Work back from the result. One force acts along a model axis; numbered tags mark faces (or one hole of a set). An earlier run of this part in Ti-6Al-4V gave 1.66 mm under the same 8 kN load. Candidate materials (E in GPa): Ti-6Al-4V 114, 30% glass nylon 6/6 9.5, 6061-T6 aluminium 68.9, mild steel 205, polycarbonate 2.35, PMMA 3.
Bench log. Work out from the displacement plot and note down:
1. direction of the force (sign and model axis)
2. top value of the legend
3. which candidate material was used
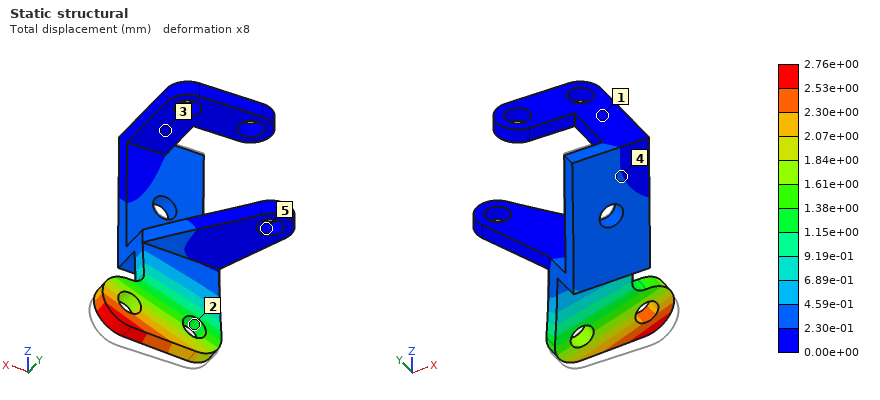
+Y
2.76e+00 mm
6061-T6 aluminium
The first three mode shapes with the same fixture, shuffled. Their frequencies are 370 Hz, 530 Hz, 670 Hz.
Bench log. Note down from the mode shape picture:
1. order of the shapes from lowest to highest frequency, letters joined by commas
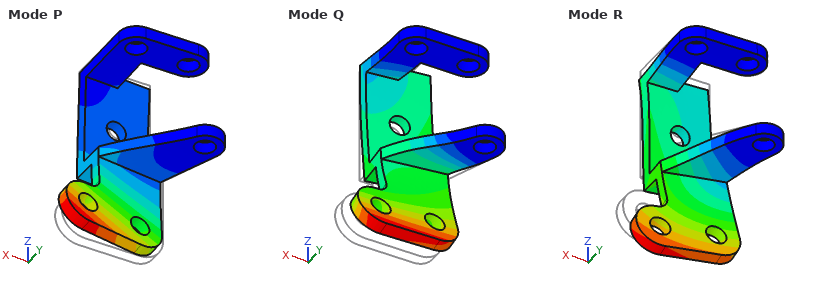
P, R, Q
